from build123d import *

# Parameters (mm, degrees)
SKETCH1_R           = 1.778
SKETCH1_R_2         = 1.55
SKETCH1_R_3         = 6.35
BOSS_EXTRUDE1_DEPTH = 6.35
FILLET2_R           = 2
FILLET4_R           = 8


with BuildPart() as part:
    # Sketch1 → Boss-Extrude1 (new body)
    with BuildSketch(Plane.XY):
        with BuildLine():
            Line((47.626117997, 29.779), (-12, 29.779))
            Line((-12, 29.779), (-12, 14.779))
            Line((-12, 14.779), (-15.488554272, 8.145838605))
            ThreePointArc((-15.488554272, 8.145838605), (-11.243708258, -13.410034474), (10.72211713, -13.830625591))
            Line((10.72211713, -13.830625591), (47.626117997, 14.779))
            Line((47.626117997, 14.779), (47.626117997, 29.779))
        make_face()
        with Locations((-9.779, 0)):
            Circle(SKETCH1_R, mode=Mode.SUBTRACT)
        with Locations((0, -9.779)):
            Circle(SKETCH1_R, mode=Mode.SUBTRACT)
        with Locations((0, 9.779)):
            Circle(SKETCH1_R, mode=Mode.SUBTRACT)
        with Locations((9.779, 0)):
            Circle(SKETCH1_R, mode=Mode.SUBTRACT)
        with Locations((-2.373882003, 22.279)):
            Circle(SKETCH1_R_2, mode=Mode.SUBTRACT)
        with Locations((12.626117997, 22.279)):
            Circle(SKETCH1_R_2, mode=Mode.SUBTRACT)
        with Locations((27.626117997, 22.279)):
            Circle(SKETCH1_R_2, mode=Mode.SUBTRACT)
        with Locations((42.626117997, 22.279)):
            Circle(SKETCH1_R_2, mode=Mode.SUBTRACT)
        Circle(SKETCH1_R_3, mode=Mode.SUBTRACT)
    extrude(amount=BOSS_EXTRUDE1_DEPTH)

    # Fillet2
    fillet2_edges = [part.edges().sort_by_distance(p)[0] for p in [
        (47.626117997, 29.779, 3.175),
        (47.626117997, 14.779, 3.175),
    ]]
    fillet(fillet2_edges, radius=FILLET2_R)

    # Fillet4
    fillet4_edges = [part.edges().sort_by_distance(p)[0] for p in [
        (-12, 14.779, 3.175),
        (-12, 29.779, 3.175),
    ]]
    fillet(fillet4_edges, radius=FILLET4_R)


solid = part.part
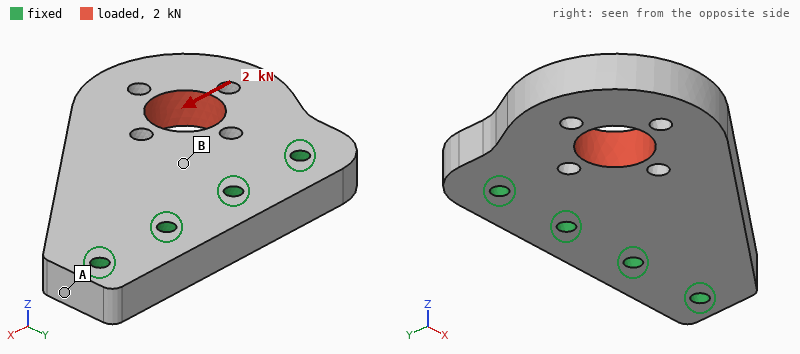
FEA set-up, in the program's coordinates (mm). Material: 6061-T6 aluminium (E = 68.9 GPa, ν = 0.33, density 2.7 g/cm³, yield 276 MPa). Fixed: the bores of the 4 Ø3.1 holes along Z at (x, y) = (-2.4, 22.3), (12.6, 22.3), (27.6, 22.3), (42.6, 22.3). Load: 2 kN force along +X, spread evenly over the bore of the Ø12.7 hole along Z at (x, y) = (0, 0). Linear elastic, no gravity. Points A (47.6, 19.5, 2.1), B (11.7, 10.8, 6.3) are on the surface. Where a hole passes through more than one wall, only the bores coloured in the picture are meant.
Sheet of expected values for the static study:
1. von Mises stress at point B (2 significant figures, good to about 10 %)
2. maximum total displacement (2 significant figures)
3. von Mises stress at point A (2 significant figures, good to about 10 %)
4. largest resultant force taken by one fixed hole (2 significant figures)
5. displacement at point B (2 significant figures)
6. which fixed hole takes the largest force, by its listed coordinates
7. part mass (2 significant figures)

13 MPa
17 µm
5.8 MPa
1.2 kN
3.5 µm
(-2.4, 22.3)
35 g
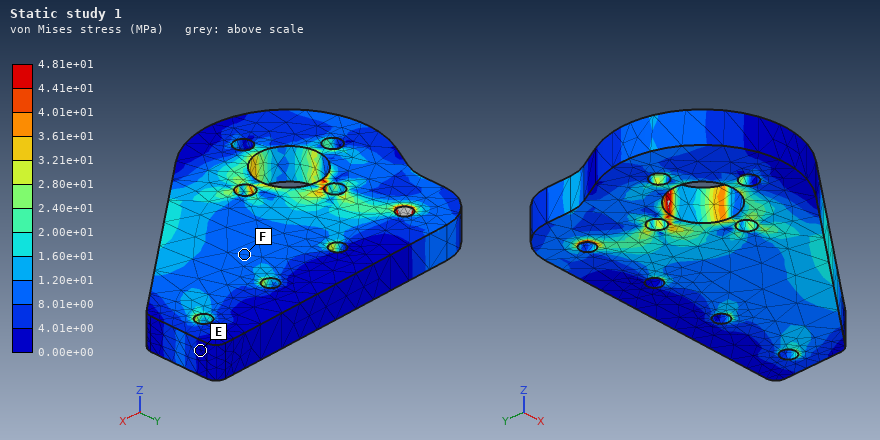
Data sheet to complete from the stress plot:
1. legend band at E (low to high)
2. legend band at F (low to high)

0.00e+00 to 4.01e+00 MPa
8.01e+00 to 1.20e+01 MPa
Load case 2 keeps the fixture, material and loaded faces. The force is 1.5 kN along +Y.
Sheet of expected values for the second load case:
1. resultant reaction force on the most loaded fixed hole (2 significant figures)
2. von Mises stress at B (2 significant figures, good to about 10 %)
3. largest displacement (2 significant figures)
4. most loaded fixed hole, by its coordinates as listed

1.1 kN
6.4 MPa
7.9 µm
(-2.4, 22.3)
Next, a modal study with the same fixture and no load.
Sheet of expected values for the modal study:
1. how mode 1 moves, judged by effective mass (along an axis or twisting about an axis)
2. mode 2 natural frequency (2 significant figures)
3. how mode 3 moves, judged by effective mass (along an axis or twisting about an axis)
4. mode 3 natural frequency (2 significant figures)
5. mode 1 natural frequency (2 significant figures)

along Z
8700 Hz
along X
15 kHz
3900 Hz
